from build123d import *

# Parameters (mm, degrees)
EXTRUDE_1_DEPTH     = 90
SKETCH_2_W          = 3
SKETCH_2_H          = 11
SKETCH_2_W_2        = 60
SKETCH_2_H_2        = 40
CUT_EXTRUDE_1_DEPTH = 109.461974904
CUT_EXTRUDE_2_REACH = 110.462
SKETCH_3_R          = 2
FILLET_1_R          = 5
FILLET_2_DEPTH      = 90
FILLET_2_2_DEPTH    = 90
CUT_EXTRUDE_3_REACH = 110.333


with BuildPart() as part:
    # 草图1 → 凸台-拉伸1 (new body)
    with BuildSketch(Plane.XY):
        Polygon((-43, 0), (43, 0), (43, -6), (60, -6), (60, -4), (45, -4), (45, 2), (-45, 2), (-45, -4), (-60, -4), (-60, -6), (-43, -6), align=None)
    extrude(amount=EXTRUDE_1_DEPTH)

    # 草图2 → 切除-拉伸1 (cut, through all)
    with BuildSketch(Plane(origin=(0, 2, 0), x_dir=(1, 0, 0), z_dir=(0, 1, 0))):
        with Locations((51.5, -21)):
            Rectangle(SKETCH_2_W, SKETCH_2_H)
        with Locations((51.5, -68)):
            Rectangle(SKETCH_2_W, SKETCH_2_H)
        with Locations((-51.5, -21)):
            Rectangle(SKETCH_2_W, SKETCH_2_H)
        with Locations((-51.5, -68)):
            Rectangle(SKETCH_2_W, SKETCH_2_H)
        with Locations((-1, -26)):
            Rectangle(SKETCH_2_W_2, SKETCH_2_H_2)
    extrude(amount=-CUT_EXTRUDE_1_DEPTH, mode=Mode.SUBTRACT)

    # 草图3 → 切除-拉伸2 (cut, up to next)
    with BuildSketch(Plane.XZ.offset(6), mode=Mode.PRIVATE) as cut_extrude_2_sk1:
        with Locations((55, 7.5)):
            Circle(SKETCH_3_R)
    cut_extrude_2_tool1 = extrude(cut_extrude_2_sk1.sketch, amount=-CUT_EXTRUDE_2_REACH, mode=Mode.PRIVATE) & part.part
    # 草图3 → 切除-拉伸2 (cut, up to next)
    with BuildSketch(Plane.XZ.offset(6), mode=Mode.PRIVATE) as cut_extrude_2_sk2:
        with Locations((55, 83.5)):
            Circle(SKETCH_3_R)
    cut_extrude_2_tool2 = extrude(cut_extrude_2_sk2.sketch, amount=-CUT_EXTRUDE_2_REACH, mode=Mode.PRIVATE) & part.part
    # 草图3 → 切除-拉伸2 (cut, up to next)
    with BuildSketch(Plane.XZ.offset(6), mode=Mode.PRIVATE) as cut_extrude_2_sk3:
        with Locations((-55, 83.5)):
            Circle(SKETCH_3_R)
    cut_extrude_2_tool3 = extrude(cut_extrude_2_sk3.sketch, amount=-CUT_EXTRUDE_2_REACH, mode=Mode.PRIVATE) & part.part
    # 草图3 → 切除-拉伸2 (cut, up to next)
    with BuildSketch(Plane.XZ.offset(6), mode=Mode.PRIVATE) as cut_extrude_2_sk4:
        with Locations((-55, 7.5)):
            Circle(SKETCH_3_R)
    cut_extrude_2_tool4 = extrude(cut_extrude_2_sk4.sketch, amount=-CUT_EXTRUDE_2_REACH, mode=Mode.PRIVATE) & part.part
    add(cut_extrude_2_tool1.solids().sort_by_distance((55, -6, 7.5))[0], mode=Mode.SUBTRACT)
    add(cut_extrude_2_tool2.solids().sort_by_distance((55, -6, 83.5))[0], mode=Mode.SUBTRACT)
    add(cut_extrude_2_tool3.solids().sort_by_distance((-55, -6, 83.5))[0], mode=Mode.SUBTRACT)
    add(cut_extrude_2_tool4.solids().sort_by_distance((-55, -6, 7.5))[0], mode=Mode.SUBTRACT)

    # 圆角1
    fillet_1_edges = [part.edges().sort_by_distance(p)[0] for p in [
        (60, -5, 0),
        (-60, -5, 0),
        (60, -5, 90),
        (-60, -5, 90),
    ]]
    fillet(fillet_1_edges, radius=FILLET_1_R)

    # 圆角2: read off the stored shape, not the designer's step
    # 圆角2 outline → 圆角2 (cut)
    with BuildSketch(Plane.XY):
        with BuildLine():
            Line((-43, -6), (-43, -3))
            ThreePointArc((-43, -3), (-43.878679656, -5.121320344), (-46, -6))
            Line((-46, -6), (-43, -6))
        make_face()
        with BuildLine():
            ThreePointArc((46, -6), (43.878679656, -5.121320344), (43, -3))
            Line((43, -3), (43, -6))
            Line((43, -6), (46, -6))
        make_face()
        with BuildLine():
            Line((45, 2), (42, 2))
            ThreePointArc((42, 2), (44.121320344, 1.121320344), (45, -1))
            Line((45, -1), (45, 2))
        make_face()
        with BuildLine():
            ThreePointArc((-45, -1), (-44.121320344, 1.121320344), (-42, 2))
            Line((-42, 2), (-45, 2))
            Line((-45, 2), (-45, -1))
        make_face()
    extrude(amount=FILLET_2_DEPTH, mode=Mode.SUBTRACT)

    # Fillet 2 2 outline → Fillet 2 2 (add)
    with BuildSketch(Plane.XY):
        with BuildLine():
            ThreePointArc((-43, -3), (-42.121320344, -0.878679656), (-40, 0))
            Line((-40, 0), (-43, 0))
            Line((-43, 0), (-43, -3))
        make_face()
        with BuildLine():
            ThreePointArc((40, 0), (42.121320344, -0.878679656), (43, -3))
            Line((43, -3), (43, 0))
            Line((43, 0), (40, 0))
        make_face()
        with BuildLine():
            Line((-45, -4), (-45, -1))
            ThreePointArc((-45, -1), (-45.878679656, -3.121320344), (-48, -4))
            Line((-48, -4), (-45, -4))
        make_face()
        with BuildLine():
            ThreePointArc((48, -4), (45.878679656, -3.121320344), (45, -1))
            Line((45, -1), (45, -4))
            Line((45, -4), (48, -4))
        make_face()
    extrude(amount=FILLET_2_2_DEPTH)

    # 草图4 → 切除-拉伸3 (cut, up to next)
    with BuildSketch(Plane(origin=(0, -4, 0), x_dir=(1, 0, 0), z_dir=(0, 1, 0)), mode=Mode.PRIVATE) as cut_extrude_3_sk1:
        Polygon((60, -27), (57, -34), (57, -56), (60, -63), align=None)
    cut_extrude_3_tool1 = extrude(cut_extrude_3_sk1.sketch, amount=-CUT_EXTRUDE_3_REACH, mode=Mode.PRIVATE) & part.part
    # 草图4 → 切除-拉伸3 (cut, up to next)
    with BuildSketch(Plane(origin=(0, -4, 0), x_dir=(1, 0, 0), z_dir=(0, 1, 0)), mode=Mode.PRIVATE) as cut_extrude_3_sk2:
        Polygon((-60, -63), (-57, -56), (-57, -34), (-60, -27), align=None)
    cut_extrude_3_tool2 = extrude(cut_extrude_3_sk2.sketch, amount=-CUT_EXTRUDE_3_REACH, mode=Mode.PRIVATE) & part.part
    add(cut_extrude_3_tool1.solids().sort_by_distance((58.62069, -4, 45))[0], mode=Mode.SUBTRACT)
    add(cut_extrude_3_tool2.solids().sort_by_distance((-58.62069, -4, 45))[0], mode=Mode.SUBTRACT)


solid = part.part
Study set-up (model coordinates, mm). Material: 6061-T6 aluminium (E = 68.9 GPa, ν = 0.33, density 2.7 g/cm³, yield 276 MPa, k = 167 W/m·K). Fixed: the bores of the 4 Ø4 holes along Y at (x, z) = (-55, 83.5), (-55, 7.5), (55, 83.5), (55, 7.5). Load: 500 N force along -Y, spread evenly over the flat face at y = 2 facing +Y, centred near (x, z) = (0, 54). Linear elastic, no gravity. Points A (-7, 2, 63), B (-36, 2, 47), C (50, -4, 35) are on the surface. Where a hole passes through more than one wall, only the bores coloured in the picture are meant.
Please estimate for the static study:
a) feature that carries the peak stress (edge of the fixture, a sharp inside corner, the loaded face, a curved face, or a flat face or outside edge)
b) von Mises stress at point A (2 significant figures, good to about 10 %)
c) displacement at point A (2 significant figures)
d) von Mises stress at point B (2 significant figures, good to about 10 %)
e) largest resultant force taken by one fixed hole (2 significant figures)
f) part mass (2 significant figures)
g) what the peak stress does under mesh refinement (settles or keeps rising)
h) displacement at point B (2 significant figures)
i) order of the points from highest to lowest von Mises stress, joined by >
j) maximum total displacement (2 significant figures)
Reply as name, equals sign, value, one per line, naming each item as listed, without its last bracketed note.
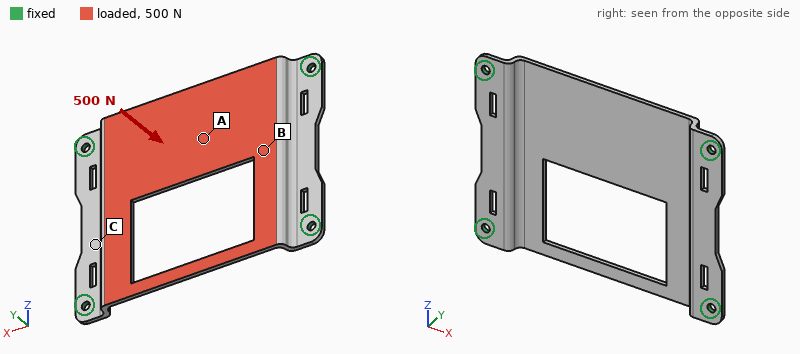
feature that carries the peak stress = edge of the fixture
von Mises stress at point A = 46 MPa
displacement at point A = 0.31 mm
von Mises stress at point B = 28 MPa
largest resultant force taken by one fixed hole = 590 N
part mass = 49 g
what the peak stress does under mesh refinement = keeps rising
displacement at point B = 0.066 mm
order of the points from highest to lowest von Mises stress, joined by > = A > B > C
maximum total displacement = 0.35 mm
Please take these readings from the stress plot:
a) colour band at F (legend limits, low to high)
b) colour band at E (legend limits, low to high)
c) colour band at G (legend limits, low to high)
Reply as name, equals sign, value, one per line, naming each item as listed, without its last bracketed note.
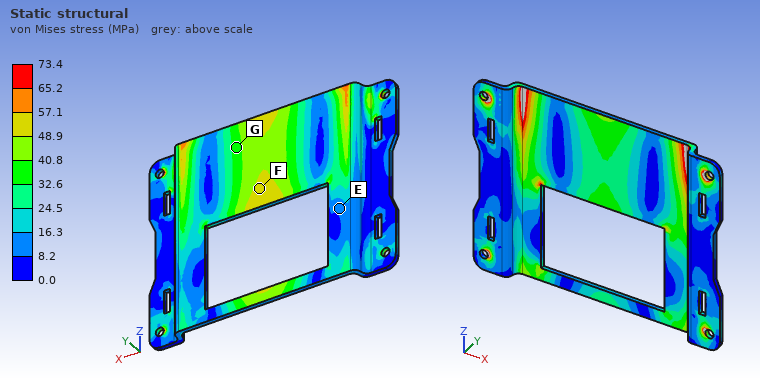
colour band at F = 48.9 to 57.1 MPa
colour band at E = 8.2 to 16.3 MPa
colour band at G = 32.6 to 40.8 MPa
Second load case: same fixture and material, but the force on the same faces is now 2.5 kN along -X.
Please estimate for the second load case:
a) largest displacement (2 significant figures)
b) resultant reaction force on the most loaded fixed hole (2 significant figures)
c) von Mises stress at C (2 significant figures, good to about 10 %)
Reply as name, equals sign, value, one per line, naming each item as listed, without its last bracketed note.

largest displacement = 0.34 mm
resultant reaction force on the most loaded fixed hole = 890 N
von Mises stress at C = 22 MPa
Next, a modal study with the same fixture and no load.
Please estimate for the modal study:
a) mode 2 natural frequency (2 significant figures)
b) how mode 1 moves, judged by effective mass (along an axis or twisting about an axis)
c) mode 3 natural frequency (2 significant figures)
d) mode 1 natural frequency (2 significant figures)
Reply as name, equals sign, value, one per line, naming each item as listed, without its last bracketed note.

mode 2 natural frequency = 1700 Hz
how mode 1 moves, judged by effective mass = along Y
mode 3 natural frequency = 1800 Hz
mode 1 natural frequency = 1400 Hz
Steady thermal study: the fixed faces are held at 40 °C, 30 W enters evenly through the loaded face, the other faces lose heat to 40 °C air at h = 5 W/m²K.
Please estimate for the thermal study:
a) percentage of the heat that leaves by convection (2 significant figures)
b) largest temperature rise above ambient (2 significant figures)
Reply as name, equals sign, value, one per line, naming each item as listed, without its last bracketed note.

percentage of the heat that leaves by convection = 4.1 %
largest temperature rise above ambient = 33 K
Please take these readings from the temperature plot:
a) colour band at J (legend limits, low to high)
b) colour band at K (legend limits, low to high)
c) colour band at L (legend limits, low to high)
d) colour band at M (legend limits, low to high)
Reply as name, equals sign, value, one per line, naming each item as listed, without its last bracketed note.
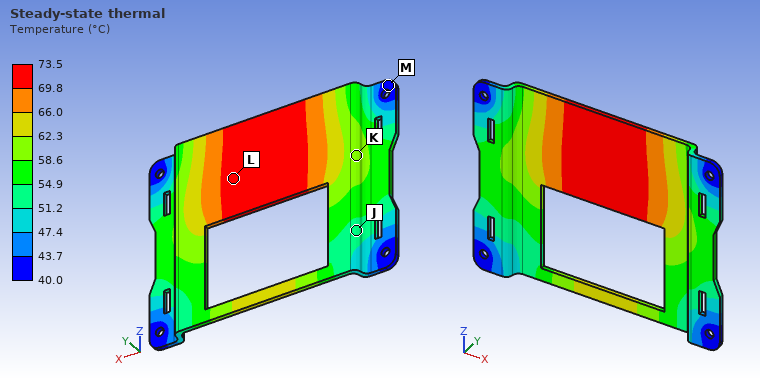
colour band at J = 51.2 to 54.9 °C
colour band at K = 58.6 to 62.3 °C
colour band at L = 69.8 to 73.5 °C
colour band at M = 40.0 to 43.7 °C
